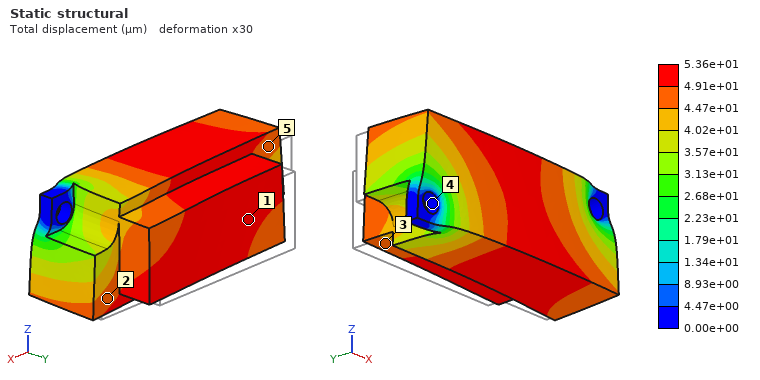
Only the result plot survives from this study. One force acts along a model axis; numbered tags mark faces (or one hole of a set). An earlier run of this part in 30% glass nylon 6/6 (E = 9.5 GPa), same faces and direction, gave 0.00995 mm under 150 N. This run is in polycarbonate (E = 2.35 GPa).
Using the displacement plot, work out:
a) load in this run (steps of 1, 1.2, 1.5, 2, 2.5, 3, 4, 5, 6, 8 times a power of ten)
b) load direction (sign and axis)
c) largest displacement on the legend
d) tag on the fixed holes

200 N
-Y
5.36e+01 µm
4
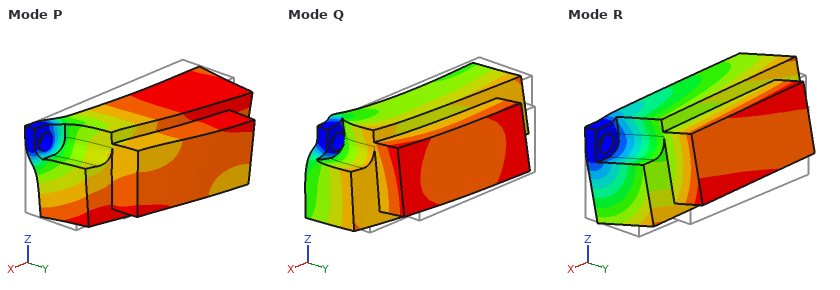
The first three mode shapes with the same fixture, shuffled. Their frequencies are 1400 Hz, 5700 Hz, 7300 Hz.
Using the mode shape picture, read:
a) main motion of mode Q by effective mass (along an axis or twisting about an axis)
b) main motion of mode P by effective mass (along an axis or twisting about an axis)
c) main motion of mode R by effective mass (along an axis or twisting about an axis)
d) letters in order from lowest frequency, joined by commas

along X
along Y
along Z
R, P, Q
